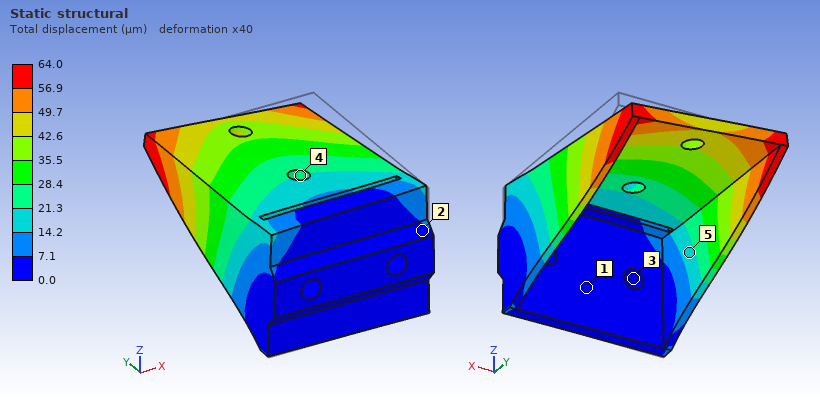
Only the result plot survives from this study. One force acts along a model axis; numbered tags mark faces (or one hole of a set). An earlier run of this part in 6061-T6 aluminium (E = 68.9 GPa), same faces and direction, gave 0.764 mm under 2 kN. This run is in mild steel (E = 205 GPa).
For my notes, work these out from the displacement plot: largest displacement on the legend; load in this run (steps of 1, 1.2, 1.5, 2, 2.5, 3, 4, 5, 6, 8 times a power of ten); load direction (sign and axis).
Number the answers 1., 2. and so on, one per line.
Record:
1. 64.0 µm
2. 500 N
3. -X
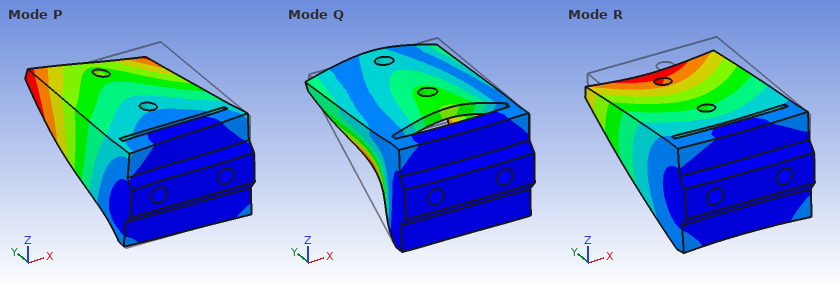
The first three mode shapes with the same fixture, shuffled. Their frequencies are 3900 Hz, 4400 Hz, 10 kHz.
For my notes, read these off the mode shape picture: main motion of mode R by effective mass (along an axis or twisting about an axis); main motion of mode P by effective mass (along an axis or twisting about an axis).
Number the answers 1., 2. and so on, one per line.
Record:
1. along Z
2. along X
